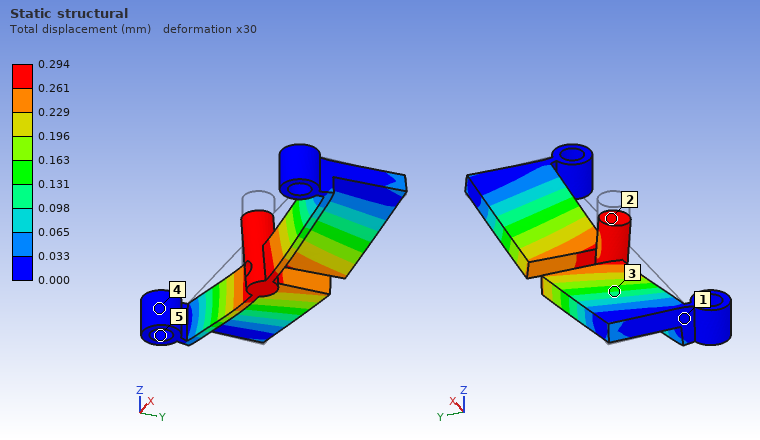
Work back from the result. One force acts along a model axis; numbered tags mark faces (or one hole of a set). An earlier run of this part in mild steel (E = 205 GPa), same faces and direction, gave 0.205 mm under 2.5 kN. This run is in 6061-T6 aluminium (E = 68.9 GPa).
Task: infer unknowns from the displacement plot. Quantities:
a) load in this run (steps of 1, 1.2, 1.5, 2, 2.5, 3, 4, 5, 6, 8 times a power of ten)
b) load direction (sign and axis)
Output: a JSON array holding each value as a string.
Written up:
["1.2 kN", "-Z"]
